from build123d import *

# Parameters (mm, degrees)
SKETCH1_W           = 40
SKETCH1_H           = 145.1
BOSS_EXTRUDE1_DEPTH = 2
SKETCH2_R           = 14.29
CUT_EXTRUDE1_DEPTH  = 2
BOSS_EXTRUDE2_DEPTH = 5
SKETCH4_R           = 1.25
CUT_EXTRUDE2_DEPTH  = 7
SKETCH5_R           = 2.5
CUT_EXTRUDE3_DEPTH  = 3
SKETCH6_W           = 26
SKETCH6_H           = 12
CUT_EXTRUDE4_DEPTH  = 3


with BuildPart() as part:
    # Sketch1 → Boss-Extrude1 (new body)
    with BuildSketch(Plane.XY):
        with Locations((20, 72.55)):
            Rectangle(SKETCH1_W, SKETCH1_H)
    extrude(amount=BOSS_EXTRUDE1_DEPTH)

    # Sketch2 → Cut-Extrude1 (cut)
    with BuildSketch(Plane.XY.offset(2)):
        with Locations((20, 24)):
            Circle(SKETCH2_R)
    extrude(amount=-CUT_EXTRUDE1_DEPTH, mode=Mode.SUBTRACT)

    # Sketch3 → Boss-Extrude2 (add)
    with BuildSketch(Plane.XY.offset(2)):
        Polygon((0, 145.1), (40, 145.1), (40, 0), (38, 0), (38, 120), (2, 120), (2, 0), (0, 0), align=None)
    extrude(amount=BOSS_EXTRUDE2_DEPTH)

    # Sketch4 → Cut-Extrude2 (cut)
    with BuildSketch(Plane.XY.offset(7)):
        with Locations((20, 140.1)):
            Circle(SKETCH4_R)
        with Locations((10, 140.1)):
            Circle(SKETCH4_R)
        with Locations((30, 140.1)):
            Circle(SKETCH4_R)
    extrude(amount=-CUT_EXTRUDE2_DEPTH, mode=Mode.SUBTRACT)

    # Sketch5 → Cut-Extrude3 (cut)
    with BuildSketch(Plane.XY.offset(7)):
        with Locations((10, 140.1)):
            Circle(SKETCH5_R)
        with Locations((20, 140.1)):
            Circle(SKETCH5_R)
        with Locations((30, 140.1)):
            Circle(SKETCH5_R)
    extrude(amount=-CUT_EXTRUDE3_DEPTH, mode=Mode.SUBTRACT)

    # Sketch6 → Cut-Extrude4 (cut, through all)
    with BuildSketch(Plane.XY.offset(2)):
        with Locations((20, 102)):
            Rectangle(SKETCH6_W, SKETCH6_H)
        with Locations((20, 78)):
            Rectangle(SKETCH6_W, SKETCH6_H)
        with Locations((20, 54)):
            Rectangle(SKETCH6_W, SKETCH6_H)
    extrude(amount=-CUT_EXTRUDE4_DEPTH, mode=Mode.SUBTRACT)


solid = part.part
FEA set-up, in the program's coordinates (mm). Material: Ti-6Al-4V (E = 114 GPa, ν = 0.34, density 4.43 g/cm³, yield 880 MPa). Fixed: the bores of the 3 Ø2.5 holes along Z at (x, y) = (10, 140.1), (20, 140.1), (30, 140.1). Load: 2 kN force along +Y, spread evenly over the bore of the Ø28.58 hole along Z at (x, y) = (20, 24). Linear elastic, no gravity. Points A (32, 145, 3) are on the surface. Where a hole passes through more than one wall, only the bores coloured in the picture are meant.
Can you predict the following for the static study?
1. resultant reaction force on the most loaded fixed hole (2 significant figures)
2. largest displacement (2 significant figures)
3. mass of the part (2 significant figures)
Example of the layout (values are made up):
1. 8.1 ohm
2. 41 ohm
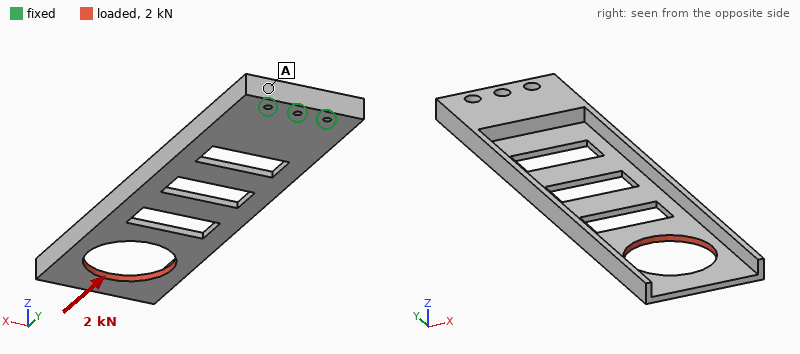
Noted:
1. 770 N
2. 0.95 mm
3. 69 g
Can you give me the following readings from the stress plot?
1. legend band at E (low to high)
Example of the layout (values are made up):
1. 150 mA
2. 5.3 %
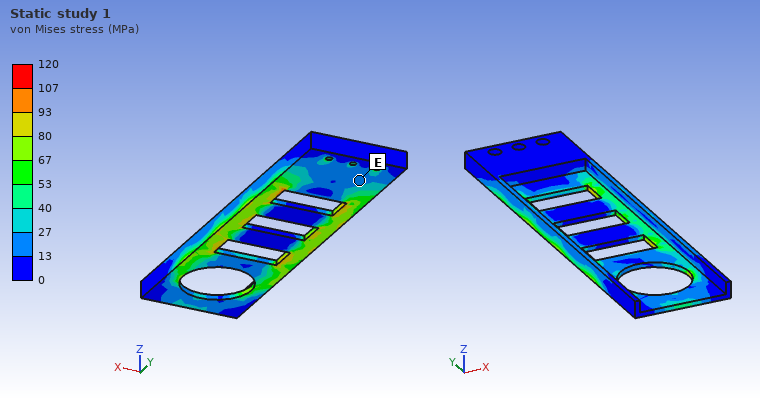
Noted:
1. 13 to 27 MPa
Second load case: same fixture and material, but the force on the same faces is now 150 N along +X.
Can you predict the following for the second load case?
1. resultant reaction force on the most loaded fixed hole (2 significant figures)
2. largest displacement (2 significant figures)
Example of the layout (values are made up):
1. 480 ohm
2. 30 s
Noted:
1. 810 N
2. 0.16 mm
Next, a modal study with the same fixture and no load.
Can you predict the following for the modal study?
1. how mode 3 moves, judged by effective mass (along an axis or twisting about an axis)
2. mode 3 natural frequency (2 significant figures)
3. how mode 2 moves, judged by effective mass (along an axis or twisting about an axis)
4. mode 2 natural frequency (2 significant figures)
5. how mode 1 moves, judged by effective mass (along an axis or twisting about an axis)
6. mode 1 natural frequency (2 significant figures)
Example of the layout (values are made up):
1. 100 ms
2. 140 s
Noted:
1. along X
2. 1500 Hz
3. twisting about Y
4. 650 Hz
5. along Z
6. 280 Hz
